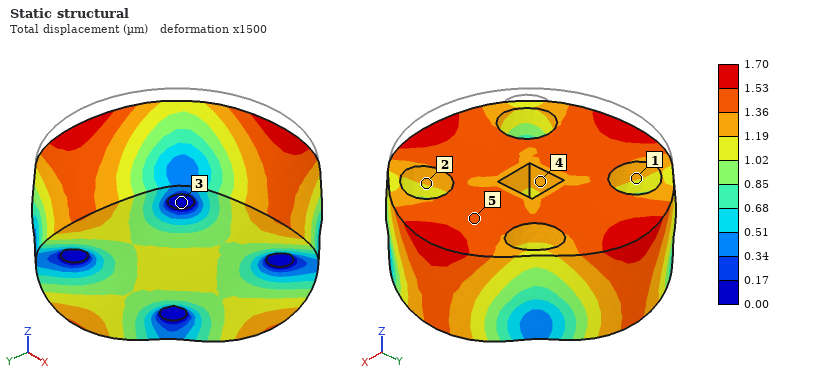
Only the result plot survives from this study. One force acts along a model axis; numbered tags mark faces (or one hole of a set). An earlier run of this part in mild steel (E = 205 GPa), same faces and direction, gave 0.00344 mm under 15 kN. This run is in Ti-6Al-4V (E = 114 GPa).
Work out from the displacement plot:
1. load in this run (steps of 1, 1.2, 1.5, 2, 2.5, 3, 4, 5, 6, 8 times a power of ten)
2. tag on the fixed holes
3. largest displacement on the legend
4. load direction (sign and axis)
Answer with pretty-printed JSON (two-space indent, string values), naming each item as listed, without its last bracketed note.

{
  "load in this run": "4 kN",
  "tag on the fixed holes": "3",
  "largest displacement on the legend": "1.70 µm",
  "load direction": "-Z"
}
